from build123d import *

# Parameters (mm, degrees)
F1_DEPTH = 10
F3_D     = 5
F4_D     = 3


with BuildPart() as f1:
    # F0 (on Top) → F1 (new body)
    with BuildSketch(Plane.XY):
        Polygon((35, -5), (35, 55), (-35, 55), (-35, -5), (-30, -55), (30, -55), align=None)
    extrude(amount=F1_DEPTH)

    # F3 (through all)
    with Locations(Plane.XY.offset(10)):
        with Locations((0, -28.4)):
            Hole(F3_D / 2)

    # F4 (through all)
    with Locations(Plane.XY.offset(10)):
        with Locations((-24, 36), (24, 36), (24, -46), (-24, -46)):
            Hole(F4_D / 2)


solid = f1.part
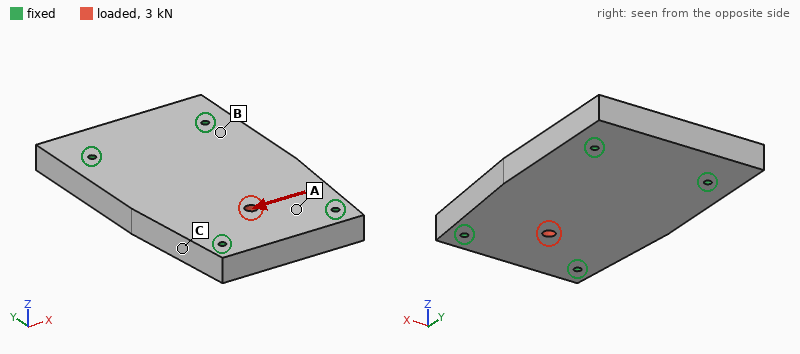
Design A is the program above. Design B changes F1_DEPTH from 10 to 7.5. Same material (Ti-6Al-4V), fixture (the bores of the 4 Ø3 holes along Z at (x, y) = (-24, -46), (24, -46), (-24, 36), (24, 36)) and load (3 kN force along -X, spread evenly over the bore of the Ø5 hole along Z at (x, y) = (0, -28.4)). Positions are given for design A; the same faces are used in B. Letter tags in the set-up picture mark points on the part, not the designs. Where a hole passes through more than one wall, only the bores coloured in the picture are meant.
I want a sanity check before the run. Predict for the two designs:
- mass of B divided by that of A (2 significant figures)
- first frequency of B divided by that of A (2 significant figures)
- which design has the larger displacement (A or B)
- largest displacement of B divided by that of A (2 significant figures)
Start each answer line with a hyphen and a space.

- 0.75
- 0.80
- B
- 1.3
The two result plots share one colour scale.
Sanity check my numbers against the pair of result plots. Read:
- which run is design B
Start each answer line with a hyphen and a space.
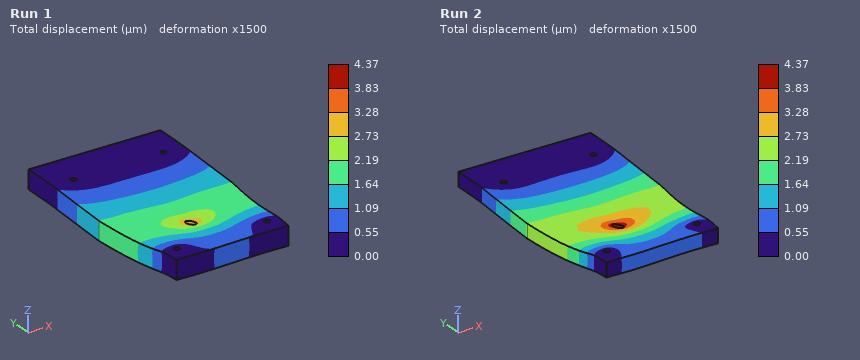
- Run 2
